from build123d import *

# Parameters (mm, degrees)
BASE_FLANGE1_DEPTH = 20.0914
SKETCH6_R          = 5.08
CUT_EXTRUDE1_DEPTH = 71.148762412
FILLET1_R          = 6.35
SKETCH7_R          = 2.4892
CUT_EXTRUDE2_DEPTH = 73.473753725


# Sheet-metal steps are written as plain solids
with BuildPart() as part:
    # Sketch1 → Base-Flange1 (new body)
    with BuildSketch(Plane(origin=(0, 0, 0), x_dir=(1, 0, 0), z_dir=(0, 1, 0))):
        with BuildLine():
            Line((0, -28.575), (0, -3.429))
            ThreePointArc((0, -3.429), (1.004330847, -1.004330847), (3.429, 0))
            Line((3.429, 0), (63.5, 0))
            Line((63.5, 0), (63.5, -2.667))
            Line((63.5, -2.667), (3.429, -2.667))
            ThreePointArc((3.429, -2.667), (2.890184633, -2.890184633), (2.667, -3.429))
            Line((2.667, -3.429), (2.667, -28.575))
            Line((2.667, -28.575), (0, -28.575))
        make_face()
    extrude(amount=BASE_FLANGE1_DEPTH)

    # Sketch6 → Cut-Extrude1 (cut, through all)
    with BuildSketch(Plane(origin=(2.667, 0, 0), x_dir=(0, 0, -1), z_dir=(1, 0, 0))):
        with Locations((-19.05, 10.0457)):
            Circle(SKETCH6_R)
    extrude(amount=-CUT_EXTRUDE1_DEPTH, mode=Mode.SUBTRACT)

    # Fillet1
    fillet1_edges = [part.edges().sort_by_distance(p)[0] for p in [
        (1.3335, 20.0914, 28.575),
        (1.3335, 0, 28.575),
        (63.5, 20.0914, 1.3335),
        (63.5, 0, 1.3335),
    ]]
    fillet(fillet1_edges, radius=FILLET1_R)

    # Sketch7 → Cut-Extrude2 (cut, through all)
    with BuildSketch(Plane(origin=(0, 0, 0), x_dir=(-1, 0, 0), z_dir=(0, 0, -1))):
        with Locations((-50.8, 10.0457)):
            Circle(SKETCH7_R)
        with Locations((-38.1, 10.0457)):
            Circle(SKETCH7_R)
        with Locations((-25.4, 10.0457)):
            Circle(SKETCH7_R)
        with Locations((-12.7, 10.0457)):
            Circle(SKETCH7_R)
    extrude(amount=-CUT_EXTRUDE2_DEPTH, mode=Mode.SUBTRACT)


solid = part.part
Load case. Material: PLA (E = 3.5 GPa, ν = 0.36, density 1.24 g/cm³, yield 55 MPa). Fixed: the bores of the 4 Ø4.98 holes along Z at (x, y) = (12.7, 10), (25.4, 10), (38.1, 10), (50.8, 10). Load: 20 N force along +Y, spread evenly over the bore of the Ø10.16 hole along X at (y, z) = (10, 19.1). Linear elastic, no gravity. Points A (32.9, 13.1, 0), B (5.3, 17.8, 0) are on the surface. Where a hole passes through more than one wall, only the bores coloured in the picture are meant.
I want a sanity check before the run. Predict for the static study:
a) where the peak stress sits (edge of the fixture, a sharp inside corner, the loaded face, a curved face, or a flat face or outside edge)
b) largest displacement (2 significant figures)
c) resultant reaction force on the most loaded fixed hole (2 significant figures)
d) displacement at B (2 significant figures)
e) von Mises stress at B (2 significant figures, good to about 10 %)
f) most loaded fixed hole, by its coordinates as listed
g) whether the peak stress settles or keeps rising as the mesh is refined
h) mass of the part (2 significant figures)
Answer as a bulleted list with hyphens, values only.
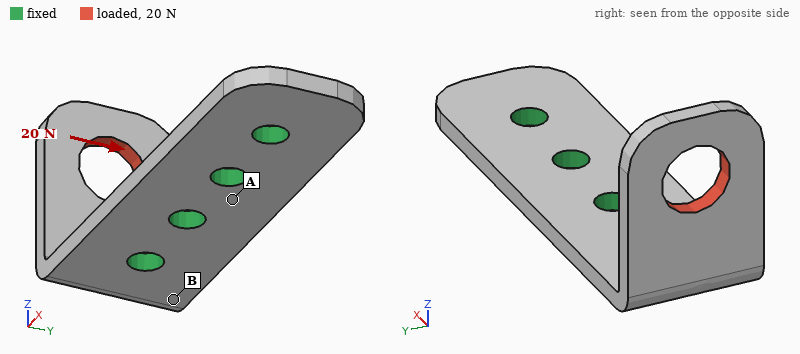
- edge of the fixture
- 0.49 mm
- 28 N
- 0.095 mm
- 5.6 MPa
- (12.7, 10)
- keeps rising
- 5.2 g
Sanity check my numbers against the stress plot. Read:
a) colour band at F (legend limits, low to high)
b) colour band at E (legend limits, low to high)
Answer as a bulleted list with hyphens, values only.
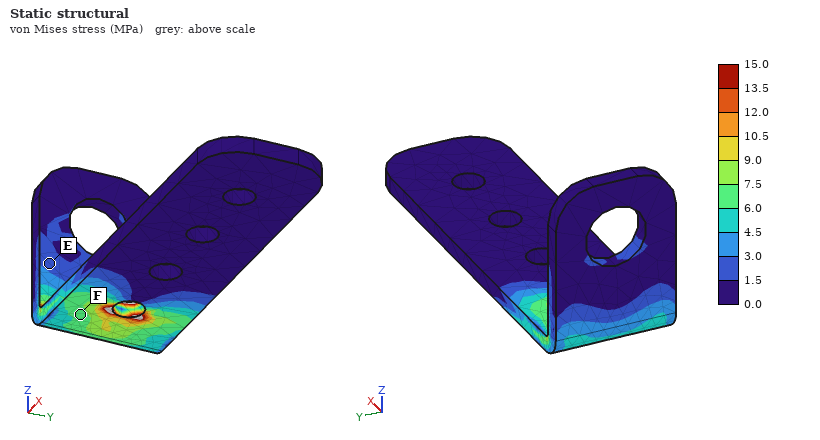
- 6.0 to 7.5 MPa
- 1.5 to 3.0 MPa
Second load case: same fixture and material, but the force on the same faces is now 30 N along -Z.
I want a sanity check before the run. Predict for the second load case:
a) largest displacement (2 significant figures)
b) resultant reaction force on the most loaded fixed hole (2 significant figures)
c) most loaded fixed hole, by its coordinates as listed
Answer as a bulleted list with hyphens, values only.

- 0.40 mm
- 35 N
- (12.7, 10)
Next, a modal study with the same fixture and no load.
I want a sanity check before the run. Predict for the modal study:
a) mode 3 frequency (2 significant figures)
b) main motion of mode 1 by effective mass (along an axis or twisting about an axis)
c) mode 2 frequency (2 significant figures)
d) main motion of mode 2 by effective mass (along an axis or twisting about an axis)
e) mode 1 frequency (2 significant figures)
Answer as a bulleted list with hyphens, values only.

- 2700 Hz
- along X
- 1100 Hz
- along Y
- 730 Hz
